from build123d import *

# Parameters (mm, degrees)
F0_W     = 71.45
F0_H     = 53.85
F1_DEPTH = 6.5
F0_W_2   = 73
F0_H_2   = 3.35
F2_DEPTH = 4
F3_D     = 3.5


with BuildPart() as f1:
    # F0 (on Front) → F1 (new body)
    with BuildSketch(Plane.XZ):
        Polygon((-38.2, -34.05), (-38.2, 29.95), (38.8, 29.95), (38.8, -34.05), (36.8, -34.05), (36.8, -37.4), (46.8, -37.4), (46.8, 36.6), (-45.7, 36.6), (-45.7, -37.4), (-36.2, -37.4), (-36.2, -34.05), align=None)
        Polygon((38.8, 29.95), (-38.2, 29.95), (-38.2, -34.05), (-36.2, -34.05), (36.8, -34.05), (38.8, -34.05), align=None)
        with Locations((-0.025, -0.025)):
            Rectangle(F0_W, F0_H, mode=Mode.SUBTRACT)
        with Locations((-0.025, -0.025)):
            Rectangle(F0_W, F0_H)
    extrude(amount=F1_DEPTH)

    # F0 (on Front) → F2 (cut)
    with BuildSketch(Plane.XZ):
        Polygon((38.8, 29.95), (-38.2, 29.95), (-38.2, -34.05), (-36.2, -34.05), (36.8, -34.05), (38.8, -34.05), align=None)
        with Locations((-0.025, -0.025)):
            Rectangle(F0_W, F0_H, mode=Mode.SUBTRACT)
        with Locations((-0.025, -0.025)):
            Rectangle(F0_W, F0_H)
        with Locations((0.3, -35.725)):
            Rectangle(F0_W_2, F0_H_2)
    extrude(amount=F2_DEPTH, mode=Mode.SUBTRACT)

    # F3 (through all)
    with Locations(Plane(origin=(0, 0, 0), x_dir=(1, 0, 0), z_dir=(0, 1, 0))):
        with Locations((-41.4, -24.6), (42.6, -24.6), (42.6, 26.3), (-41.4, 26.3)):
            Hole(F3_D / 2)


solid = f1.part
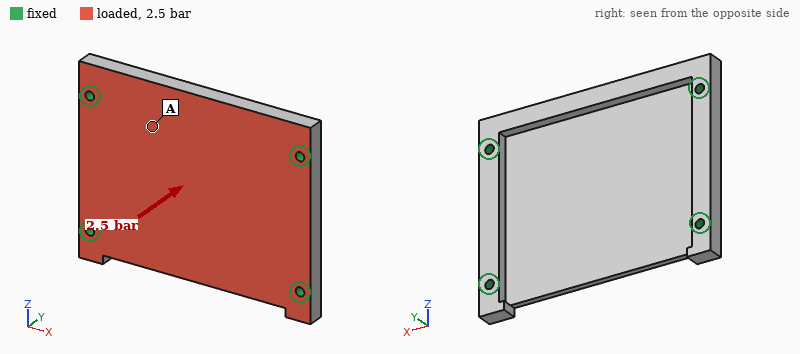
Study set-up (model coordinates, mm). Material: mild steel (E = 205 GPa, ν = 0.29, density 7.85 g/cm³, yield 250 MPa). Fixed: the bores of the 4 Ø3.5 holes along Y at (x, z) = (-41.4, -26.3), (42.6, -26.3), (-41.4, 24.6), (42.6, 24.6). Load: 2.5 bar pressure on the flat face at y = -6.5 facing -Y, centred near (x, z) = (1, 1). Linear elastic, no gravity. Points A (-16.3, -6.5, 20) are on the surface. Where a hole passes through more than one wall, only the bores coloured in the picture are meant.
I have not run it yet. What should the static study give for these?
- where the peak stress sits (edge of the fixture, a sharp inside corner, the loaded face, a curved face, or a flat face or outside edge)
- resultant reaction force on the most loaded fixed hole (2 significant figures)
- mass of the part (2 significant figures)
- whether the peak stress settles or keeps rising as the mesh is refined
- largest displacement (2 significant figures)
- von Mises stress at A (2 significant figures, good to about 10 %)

edge of the fixture
480 N
180 g
keeps rising
0.11 mm
26 MPa
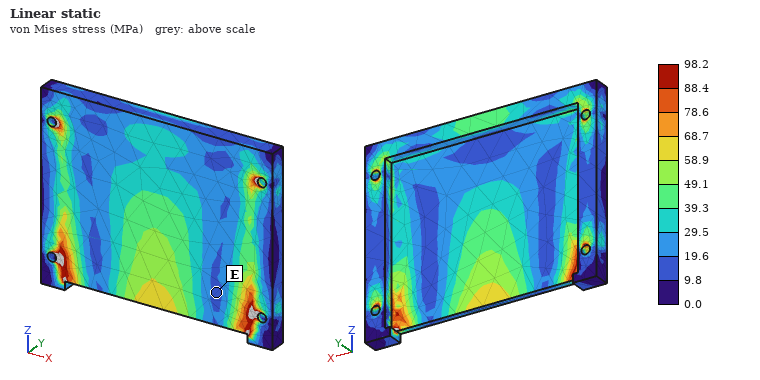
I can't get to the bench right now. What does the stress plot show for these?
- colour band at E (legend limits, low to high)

9.8 to 19.6 MPa
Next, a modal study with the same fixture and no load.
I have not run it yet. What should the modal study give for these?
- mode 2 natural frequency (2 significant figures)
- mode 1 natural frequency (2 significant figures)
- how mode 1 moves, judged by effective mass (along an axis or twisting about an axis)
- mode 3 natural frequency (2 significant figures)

3400 Hz
2200 Hz
along Y
4900 Hz
